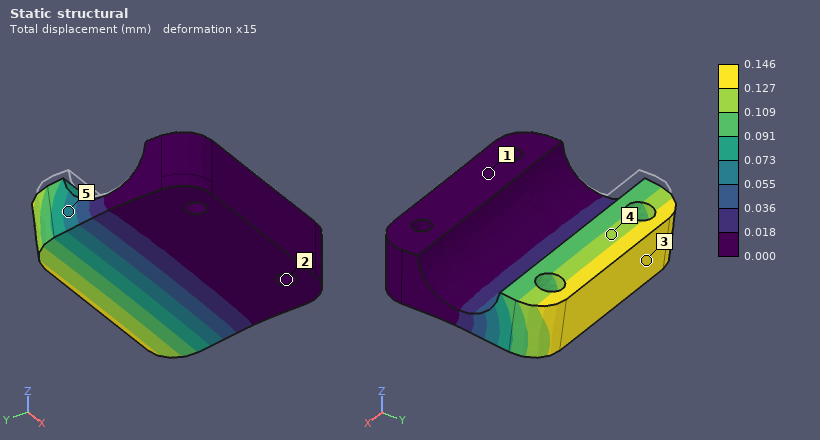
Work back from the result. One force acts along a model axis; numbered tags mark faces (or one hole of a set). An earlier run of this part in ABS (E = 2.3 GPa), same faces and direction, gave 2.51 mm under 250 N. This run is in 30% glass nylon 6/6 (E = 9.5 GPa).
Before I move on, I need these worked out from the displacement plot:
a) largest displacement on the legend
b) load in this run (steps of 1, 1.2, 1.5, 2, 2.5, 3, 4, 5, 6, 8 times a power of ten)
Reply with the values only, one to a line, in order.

0.146 mm
60 N
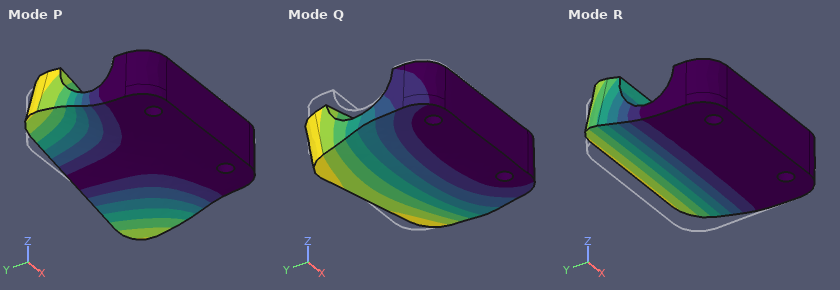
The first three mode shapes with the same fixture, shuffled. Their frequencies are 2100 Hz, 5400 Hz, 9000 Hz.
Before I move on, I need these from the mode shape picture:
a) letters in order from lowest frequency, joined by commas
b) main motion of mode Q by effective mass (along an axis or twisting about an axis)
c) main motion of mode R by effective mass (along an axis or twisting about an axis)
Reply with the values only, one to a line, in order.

R, P, Q
along X
along Z
